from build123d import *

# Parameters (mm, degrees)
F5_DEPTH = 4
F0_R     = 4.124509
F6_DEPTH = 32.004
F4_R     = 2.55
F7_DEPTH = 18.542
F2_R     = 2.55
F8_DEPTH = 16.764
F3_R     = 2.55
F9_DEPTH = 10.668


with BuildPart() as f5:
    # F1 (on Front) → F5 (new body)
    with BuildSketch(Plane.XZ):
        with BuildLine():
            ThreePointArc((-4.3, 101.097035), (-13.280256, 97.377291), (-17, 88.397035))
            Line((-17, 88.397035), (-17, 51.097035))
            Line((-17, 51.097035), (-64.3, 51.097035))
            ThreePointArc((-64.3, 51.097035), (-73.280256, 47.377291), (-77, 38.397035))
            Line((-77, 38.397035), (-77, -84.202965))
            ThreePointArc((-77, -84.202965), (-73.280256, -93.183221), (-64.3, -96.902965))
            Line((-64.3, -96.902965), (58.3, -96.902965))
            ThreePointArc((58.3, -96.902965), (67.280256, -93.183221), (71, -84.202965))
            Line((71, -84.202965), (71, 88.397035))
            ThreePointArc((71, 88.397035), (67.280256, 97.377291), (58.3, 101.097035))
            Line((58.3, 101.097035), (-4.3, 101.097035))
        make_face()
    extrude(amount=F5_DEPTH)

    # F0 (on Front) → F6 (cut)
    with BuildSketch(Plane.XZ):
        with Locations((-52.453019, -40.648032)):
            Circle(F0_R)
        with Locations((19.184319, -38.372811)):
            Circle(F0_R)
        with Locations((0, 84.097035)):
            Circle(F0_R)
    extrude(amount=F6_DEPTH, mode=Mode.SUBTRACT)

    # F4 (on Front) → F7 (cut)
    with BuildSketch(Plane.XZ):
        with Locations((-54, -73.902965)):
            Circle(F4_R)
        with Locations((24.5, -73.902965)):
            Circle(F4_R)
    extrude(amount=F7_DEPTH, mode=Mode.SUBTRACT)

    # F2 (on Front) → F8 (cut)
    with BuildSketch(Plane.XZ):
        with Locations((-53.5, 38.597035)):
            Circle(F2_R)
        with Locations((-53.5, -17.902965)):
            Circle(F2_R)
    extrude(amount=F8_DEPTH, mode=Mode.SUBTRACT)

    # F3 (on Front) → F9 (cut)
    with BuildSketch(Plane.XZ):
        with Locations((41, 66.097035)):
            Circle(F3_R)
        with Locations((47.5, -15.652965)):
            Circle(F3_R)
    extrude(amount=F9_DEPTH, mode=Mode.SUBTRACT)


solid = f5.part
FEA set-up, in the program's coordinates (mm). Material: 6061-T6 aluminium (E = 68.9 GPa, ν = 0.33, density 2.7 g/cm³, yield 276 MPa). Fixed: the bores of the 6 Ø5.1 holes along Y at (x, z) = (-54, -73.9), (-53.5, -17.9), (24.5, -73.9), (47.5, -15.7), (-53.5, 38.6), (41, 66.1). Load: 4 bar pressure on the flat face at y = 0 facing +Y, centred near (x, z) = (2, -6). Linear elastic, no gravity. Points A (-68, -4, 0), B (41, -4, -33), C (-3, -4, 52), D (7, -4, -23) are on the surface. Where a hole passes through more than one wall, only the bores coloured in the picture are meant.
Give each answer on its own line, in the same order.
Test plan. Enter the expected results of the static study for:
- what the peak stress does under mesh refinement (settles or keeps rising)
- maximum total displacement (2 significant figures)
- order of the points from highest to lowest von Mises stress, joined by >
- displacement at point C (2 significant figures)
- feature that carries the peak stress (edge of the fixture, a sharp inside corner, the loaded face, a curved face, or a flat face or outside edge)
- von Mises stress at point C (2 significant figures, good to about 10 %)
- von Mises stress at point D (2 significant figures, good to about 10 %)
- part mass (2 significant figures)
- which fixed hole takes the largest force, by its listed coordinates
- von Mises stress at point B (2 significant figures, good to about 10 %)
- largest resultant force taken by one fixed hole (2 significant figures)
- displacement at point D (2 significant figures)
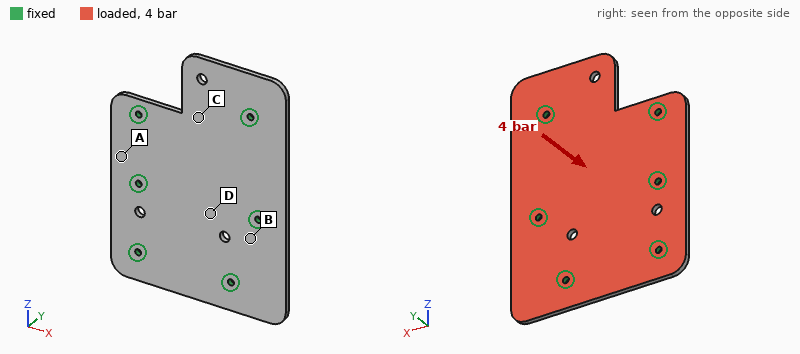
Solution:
keeps rising
0.91 mm
C > B > D > A
0.42 mm
edge of the fixture
88 MPa
43 MPa
280 g
(41, 66.1)
62 MPa
2.4 kN
0.25 mm
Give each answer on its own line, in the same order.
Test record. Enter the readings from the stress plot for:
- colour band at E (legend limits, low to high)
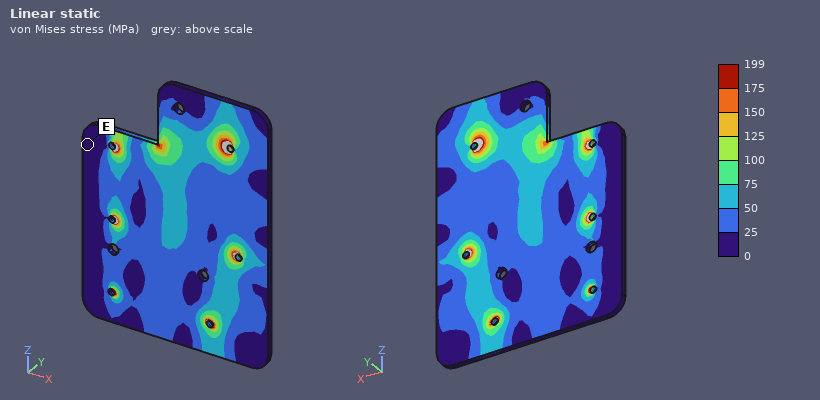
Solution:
0 to 25 MPa
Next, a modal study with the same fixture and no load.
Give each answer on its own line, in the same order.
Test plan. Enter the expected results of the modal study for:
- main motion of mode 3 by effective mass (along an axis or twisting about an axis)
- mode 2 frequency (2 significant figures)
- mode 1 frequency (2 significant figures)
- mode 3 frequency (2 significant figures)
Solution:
along Y
1800 Hz
1300 Hz
1900 Hz
